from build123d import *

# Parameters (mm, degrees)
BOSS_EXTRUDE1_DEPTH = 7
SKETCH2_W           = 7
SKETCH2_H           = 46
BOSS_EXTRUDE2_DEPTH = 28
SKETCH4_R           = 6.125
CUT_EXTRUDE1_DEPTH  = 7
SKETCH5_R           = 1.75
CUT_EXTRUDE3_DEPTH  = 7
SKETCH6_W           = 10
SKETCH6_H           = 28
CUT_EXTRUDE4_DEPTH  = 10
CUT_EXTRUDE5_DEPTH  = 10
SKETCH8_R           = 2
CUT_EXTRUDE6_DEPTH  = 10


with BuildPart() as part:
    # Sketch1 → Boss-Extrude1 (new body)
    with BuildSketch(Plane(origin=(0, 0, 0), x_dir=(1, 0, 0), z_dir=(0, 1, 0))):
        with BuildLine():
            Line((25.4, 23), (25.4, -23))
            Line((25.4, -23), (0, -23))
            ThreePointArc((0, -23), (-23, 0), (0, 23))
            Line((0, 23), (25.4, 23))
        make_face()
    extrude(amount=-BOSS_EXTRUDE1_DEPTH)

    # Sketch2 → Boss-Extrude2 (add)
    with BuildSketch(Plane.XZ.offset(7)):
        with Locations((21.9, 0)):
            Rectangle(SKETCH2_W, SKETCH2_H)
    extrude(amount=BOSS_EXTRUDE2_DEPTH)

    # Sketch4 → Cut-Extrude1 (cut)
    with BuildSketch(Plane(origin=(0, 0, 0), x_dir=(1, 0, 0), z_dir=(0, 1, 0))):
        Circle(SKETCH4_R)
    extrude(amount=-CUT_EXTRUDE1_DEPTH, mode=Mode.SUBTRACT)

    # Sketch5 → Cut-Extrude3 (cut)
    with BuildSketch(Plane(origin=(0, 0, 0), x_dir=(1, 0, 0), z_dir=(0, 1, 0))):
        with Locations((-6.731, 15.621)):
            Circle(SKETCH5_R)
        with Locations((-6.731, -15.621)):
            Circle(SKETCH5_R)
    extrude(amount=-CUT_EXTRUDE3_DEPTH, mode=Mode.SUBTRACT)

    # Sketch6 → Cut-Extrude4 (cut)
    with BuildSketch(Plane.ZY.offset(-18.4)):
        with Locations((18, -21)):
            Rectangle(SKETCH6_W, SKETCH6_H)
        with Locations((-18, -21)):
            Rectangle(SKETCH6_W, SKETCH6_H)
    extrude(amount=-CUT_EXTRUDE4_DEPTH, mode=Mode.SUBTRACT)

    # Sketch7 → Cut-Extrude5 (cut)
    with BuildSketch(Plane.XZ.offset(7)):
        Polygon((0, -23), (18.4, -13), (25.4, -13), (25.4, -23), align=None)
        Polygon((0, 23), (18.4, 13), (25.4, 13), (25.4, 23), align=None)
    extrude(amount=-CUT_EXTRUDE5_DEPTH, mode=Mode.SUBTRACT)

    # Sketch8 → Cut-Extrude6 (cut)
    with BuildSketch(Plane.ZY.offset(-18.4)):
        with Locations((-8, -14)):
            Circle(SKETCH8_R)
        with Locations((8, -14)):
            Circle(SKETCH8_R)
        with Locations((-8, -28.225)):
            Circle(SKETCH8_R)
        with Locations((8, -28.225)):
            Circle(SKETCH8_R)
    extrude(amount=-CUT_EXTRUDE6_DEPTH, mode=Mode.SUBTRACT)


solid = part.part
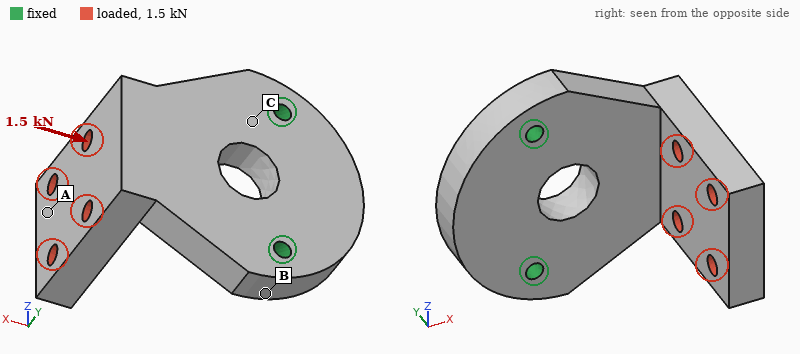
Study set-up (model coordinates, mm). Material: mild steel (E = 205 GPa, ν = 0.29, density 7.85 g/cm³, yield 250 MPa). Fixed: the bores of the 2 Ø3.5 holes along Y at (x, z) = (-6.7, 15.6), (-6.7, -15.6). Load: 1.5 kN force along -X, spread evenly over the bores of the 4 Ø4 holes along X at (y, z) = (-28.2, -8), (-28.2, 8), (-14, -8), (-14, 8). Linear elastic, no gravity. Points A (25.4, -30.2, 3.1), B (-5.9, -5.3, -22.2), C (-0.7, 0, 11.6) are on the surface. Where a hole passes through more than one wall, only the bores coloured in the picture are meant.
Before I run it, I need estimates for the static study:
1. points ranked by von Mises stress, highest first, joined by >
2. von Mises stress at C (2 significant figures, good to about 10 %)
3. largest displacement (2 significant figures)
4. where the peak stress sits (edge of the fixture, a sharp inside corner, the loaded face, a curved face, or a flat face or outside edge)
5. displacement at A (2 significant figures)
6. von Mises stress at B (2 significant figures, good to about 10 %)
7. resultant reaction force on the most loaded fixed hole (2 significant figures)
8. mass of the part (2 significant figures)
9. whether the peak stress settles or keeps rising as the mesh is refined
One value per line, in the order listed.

C > B > A
91 MPa
0.20 mm
edge of the fixture
0.17 mm
44 MPa
780 N
120 g
keeps rising
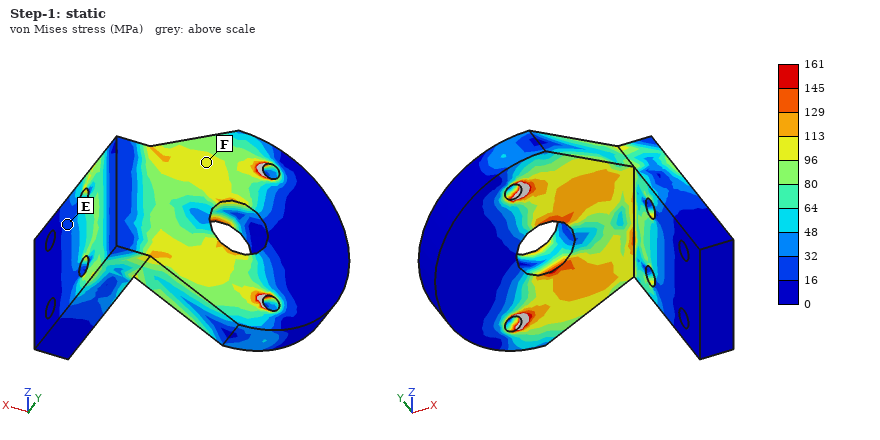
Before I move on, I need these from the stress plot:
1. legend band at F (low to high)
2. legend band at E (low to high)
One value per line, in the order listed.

96 to 113 MPa
16 to 32 MPa
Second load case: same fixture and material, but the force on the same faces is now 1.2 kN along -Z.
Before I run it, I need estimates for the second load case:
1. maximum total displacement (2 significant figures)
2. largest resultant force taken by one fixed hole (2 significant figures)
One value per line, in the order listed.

56 µm
1.3 kN
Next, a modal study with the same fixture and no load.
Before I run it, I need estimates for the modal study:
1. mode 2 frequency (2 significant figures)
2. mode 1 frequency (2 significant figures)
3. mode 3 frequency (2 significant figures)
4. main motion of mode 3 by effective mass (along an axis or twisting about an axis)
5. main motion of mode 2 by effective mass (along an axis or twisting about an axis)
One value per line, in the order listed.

4400 Hz
2200 Hz
5800 Hz
along Y
along Z
